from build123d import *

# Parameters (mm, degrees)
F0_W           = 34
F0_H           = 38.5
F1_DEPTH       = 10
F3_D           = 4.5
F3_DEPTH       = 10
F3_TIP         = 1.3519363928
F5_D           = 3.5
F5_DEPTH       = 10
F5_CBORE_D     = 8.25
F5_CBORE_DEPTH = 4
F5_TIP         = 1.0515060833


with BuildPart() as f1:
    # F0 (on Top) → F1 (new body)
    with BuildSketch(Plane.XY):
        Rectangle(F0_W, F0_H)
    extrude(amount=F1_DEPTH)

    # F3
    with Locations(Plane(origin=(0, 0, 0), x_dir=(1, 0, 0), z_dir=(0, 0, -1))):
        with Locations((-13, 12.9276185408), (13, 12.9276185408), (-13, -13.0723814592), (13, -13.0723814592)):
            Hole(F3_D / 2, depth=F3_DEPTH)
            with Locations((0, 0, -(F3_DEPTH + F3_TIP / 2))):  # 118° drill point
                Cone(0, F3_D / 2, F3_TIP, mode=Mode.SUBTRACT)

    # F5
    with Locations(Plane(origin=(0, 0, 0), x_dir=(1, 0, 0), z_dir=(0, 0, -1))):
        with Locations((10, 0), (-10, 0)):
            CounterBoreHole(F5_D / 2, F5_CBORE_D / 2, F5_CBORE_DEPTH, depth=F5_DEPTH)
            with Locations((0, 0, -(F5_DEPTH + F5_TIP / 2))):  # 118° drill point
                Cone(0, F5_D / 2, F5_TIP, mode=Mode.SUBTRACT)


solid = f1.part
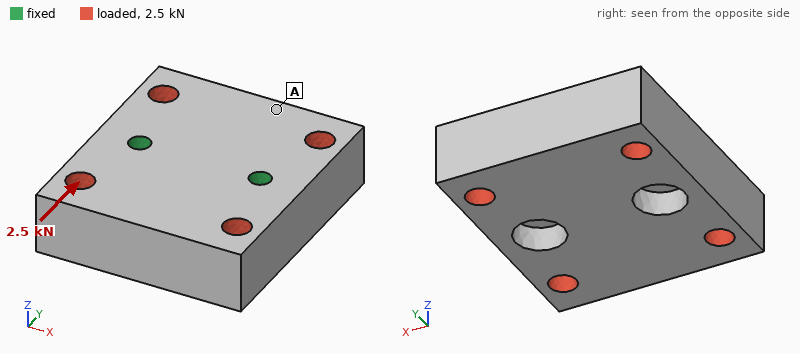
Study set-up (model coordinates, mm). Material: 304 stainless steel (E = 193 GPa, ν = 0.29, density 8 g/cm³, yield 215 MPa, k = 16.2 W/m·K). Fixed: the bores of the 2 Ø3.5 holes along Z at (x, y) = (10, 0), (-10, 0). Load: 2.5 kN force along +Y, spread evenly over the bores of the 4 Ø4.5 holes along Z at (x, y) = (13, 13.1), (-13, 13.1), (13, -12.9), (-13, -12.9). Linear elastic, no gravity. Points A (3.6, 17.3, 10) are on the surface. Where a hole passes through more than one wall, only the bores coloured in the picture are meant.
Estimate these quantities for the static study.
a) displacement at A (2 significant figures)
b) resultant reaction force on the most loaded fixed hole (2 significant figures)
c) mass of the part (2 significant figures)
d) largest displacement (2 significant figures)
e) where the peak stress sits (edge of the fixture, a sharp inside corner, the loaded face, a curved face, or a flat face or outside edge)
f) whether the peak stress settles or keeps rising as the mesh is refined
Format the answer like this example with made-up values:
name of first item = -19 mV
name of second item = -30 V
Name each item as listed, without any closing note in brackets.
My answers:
displacement at A = 2.2 µm
resultant reaction force on the most loaded fixed hole = 1.3 kN
mass of the part = 95 g
largest displacement = 3.0 µm
where the peak stress sits = edge of the fixture
whether the peak stress settles or keeps rising as the mesh is refined = keeps rising
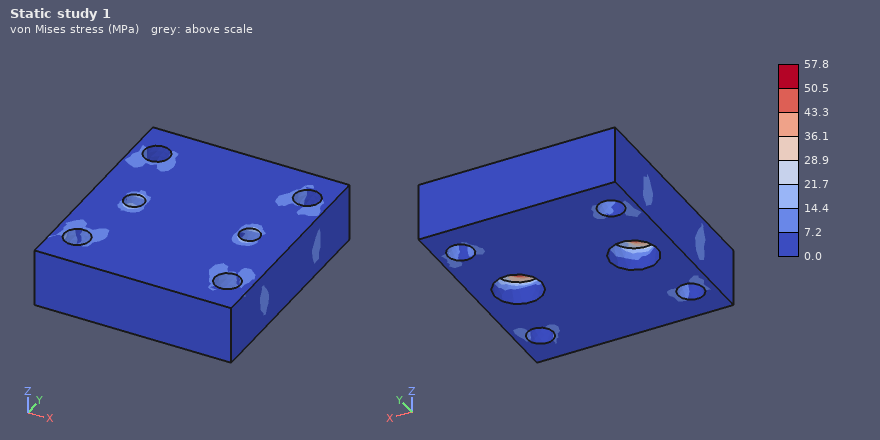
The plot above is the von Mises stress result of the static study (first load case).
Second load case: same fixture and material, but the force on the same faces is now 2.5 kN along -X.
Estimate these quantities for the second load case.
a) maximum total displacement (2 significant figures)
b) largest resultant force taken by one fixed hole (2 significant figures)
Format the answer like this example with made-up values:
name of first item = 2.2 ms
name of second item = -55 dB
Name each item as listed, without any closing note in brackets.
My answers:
maximum total displacement = 1.7 µm
largest resultant force taken by one fixed hole = 1.3 kN
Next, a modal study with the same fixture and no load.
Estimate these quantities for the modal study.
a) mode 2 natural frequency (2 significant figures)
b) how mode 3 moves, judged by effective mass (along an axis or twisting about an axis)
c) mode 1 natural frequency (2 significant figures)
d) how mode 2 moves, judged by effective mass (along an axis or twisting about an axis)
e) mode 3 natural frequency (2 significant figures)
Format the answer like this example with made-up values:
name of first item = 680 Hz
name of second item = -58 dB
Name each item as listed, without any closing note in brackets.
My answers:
mode 2 natural frequency = 16 kHz
how mode 3 moves, judged by effective mass = twisting about Z
mode 1 natural frequency = 8700 Hz
how mode 2 moves, judged by effective mass = along Z
mode 3 natural frequency = 20 kHz
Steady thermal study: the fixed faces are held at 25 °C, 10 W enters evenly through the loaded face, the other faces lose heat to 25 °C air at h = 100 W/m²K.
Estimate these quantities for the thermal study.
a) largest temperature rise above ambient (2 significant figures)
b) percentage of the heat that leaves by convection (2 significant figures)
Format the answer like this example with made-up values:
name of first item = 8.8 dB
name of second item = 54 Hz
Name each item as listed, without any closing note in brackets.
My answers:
largest temperature rise above ambient = 16 K
percentage of the heat that leaves by convection = 39 %
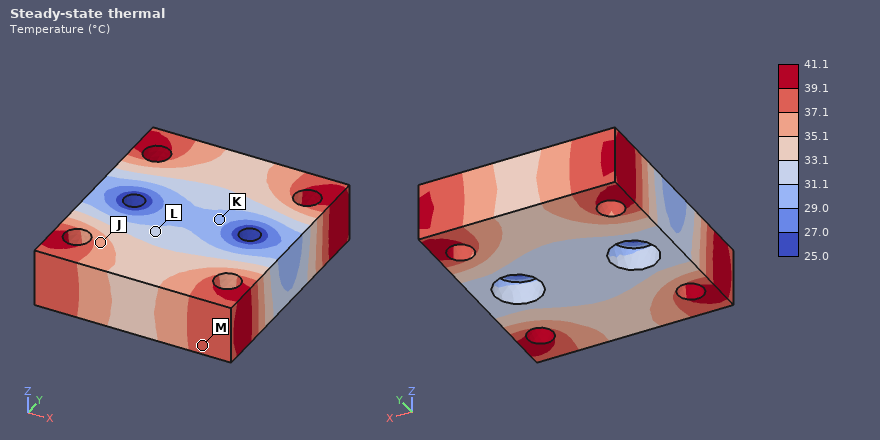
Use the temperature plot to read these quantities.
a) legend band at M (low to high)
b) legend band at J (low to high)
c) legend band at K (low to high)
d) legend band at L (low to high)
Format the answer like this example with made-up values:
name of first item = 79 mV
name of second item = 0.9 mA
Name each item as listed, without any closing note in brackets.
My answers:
legend band at M = 37.1 to 39.1 °C
legend band at J = 35.1 to 37.1 °C
legend band at K = 29.0 to 31.1 °C
legend band at L = 31.1 to 33.1 °C
